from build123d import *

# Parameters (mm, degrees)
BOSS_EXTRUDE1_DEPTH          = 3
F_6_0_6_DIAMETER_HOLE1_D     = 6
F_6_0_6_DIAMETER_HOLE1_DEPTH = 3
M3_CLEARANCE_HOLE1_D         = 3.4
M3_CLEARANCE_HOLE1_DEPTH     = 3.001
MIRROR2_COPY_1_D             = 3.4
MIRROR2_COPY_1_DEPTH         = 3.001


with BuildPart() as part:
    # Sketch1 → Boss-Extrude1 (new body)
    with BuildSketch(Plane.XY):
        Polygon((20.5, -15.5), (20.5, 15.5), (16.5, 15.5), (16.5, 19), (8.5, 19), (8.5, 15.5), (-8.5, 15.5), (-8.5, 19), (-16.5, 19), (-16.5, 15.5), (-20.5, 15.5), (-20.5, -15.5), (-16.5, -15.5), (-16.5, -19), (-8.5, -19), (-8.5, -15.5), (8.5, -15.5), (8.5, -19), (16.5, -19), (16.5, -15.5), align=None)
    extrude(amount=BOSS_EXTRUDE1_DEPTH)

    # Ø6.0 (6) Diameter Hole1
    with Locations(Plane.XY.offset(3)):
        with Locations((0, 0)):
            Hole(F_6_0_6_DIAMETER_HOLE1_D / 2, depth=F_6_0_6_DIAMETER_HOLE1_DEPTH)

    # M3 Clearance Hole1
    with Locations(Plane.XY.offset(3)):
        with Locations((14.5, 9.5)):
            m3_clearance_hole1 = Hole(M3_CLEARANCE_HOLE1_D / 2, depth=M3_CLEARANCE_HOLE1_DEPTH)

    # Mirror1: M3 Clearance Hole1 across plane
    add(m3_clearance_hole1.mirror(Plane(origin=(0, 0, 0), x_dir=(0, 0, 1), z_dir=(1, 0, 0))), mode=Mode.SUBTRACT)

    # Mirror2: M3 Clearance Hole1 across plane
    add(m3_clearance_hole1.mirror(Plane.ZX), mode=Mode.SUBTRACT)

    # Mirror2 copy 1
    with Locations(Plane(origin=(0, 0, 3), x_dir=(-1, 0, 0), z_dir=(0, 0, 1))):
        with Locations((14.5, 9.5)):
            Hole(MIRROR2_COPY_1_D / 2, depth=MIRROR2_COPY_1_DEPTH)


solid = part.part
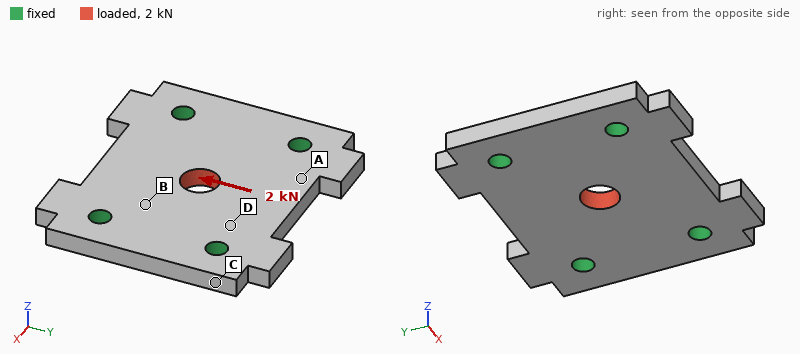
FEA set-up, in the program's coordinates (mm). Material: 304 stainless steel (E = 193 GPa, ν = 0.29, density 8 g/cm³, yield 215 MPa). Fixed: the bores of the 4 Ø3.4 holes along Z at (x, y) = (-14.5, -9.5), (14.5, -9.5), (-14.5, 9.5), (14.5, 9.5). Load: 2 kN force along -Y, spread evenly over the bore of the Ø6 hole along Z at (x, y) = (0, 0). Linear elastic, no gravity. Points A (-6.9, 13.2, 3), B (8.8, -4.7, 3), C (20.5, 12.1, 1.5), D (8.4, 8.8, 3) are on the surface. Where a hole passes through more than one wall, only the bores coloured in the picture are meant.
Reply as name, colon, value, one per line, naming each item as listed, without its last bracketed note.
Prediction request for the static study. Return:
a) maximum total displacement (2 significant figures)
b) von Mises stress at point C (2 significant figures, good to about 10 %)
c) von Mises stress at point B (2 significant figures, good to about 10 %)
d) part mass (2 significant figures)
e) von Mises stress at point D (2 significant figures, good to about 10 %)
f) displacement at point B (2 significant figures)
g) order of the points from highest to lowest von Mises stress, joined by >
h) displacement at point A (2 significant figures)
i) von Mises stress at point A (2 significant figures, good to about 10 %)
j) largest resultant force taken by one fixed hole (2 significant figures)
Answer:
maximum total displacement: 2.8 µm
von Mises stress at point C: 5.8 MPa
von Mises stress at point B: 24 MPa
part mass: 32 g
von Mises stress at point D: 20 MPa
displacement at point B: 1.0 µm
order of the points from highest to lowest von Mises stress, joined by >: B > D > A > C
displacement at point A: 1.3 µm
von Mises stress at point A: 12 MPa
largest resultant force taken by one fixed hole: 580 N
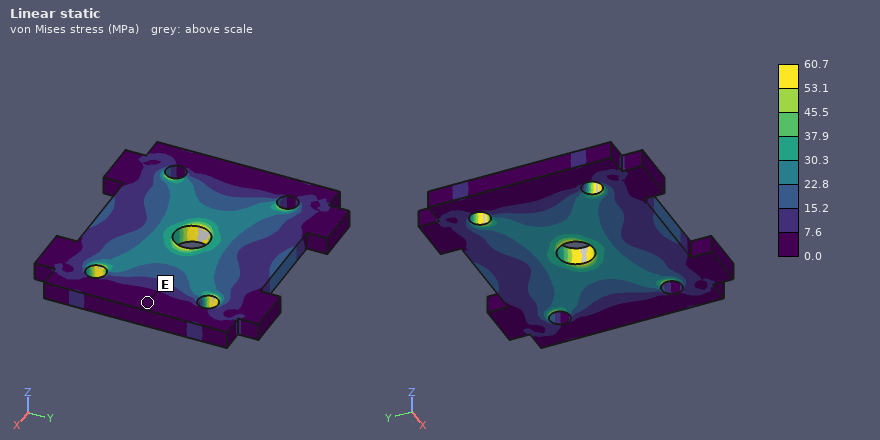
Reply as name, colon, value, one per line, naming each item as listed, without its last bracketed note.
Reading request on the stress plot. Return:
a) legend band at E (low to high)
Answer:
legend band at E: 0.0 to 7.6 MPa
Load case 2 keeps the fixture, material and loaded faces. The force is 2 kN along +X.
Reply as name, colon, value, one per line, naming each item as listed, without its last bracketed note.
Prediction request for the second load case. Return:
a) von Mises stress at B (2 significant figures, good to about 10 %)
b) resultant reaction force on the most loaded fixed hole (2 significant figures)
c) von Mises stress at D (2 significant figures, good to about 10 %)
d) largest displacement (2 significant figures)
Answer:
von Mises stress at B: 20 MPa
resultant reaction force on the most loaded fixed hole: 530 N
von Mises stress at D: 16 MPa
largest displacement: 1.8 µm
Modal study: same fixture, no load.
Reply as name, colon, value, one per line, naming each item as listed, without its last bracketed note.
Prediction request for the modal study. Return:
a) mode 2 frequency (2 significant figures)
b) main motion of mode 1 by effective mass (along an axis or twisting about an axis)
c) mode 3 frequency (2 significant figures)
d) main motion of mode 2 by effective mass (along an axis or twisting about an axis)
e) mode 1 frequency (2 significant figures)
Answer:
mode 2 frequency: 20 kHz
main motion of mode 1 by effective mass: along Z
mode 3 frequency: 25 kHz
main motion of mode 2 by effective mass: twisting about X
mode 1 frequency: 17 kHz
